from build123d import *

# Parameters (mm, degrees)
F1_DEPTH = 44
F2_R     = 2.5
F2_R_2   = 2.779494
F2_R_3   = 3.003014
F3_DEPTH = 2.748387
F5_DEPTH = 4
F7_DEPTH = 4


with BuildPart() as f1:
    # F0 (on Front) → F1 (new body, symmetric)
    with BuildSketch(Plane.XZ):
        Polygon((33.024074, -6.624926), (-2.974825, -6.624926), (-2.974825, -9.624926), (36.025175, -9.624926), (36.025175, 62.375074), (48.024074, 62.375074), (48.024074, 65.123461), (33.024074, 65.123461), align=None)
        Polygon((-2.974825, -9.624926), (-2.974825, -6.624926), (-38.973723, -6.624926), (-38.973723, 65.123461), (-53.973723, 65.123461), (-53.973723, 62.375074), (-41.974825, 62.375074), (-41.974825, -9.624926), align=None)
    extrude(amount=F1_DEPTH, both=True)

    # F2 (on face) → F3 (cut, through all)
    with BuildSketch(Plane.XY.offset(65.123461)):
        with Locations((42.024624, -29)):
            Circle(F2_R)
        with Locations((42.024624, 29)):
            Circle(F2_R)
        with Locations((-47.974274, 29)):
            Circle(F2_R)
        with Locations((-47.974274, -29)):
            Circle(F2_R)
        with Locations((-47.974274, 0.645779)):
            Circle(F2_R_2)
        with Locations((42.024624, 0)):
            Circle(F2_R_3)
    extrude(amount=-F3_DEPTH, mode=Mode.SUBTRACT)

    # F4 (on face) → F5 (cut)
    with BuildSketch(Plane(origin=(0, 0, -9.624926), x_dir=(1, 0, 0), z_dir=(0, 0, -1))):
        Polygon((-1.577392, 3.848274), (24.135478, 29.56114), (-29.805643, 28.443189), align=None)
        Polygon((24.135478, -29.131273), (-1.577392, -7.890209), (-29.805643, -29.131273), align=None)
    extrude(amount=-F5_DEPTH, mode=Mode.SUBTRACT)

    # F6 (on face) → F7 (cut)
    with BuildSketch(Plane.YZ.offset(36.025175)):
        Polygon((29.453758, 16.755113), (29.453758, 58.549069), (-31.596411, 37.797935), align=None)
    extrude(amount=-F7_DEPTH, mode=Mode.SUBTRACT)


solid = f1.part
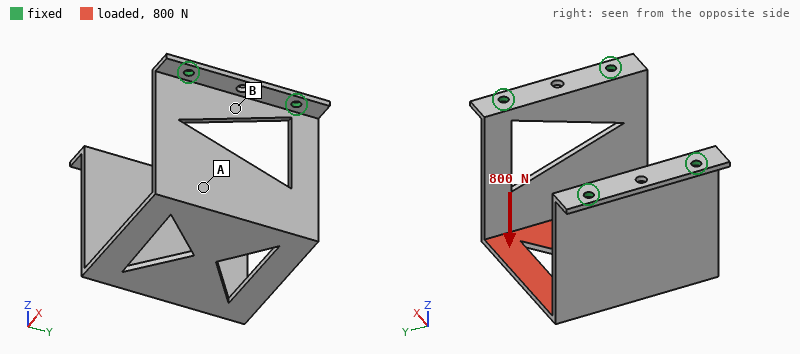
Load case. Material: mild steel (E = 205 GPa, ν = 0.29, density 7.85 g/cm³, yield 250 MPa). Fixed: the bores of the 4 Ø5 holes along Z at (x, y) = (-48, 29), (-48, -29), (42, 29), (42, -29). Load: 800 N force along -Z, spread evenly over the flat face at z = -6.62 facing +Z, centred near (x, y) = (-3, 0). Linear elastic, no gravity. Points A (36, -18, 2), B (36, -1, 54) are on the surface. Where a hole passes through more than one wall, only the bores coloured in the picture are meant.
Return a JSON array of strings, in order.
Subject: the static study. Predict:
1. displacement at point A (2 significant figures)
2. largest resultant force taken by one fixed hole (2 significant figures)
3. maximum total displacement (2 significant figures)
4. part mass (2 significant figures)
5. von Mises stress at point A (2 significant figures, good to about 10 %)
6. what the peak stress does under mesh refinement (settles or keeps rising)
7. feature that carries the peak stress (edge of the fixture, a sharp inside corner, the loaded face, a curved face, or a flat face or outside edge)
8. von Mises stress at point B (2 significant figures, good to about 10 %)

["26 µm", "220 N", "70 µm", "440 g", "19 MPa", "keeps rising", "a sharp inside corner", "5.5 MPa"]
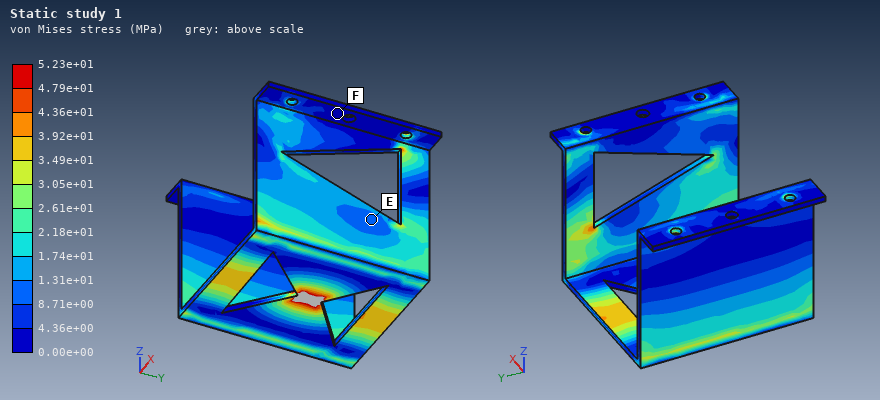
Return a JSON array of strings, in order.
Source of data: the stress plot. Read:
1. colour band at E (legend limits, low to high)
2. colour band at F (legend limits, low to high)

["8.71e+00 to 1.31e+01 MPa", "0.00e+00 to 4.36e+00 MPa"]
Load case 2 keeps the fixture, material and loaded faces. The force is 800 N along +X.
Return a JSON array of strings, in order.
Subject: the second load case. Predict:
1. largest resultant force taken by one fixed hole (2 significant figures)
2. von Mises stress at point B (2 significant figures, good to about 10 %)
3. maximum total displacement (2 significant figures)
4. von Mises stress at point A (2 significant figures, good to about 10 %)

["340 N", "40 MPa", "0.65 mm", "73 MPa"]
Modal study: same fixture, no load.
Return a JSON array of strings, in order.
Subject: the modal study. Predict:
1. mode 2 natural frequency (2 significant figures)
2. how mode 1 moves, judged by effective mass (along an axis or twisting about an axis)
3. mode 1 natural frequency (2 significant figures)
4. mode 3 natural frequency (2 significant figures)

["1500 Hz", "along X", "370 Hz", "1500 Hz"]
